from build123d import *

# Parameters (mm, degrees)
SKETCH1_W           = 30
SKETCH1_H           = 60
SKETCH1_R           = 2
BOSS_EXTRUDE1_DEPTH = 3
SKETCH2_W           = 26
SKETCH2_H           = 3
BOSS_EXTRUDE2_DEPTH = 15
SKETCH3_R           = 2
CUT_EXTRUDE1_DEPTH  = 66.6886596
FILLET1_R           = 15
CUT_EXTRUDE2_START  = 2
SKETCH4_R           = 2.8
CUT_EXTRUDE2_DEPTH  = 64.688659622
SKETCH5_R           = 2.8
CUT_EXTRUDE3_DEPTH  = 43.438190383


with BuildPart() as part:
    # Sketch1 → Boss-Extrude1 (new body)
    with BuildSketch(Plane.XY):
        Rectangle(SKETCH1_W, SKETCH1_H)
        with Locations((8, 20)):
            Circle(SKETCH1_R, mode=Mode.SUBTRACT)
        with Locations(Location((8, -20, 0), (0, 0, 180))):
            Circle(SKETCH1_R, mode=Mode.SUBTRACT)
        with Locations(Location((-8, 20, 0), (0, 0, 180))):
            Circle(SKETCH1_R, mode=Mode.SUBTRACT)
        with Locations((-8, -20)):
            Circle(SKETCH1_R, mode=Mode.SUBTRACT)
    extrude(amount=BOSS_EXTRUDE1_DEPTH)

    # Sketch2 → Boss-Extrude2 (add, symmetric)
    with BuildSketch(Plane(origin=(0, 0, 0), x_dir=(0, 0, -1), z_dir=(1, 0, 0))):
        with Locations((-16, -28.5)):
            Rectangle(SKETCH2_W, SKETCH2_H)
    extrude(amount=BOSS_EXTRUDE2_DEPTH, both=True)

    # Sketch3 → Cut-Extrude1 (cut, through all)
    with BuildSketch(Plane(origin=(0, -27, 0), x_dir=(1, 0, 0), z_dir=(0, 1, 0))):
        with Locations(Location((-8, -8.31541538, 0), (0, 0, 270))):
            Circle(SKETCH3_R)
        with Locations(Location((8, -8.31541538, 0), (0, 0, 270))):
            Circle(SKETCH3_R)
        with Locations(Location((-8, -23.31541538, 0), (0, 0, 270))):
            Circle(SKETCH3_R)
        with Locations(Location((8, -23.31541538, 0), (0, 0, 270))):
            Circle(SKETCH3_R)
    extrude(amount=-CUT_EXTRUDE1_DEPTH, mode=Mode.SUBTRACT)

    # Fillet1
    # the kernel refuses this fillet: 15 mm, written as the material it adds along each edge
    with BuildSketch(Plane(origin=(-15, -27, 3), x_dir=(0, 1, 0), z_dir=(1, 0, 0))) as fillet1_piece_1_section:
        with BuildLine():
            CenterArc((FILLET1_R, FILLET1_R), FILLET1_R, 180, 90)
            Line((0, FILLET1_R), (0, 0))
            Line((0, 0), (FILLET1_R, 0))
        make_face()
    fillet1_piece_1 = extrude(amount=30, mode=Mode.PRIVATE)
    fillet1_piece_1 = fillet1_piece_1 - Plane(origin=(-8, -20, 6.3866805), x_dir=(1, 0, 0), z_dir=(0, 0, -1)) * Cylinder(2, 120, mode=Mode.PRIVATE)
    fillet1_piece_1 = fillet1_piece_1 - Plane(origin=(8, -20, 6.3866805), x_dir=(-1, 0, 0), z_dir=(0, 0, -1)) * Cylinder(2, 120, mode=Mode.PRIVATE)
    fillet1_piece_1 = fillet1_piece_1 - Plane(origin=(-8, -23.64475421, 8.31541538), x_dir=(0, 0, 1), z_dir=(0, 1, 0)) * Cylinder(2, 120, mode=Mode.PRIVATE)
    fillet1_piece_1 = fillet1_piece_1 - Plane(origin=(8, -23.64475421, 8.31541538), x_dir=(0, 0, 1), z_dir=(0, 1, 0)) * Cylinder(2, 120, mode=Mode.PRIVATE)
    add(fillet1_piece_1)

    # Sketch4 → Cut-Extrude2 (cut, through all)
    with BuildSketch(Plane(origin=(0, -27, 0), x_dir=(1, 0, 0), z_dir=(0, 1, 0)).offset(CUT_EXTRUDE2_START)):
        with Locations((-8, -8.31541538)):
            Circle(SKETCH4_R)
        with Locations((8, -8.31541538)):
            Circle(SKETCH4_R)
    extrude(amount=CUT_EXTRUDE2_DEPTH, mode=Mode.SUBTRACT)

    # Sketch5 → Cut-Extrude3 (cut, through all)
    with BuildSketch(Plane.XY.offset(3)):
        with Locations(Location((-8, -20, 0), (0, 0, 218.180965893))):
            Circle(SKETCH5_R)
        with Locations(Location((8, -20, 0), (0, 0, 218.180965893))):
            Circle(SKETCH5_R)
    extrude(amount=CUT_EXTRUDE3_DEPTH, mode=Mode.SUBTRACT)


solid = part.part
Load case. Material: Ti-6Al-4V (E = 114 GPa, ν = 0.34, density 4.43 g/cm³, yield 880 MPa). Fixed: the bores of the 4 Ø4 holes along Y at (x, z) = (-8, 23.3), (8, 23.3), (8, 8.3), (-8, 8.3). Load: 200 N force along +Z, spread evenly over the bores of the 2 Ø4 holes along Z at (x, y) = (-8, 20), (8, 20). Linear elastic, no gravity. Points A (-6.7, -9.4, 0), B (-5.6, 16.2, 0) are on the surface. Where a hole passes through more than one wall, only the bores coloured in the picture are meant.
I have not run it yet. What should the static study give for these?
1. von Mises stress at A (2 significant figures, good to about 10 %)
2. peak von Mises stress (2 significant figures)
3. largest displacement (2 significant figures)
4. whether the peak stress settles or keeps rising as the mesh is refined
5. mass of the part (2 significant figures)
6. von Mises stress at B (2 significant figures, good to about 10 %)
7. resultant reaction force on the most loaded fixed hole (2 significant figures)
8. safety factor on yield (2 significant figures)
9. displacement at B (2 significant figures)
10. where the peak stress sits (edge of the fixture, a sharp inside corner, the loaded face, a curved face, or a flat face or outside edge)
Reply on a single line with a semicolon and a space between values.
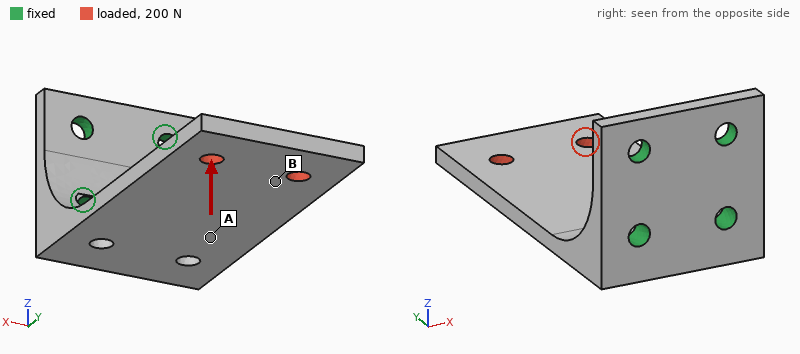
120 MPa; 160 MPa; 0.71 mm; settles; 38 g; 22 MPa; 140 N; 5.4; 0.45 mm; a curved face
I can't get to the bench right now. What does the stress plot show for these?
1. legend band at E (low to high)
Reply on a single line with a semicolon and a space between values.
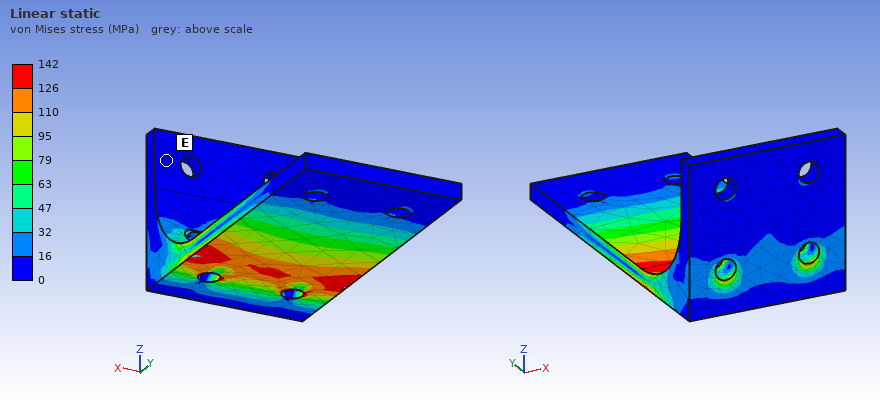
0 to 16 MPa
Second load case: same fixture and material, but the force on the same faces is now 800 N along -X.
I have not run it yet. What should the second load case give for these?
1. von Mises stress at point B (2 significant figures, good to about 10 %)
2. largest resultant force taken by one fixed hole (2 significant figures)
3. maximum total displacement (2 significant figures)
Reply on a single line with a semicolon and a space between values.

21 MPa; 2.0 kN; 0.10 mm
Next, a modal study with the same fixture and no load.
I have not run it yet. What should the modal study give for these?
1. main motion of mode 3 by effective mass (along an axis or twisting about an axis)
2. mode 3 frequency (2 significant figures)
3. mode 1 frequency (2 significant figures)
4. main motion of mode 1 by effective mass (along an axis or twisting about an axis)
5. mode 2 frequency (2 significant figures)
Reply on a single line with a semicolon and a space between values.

along X; 5100 Hz; 1000 Hz; along Z; 3500 Hz
